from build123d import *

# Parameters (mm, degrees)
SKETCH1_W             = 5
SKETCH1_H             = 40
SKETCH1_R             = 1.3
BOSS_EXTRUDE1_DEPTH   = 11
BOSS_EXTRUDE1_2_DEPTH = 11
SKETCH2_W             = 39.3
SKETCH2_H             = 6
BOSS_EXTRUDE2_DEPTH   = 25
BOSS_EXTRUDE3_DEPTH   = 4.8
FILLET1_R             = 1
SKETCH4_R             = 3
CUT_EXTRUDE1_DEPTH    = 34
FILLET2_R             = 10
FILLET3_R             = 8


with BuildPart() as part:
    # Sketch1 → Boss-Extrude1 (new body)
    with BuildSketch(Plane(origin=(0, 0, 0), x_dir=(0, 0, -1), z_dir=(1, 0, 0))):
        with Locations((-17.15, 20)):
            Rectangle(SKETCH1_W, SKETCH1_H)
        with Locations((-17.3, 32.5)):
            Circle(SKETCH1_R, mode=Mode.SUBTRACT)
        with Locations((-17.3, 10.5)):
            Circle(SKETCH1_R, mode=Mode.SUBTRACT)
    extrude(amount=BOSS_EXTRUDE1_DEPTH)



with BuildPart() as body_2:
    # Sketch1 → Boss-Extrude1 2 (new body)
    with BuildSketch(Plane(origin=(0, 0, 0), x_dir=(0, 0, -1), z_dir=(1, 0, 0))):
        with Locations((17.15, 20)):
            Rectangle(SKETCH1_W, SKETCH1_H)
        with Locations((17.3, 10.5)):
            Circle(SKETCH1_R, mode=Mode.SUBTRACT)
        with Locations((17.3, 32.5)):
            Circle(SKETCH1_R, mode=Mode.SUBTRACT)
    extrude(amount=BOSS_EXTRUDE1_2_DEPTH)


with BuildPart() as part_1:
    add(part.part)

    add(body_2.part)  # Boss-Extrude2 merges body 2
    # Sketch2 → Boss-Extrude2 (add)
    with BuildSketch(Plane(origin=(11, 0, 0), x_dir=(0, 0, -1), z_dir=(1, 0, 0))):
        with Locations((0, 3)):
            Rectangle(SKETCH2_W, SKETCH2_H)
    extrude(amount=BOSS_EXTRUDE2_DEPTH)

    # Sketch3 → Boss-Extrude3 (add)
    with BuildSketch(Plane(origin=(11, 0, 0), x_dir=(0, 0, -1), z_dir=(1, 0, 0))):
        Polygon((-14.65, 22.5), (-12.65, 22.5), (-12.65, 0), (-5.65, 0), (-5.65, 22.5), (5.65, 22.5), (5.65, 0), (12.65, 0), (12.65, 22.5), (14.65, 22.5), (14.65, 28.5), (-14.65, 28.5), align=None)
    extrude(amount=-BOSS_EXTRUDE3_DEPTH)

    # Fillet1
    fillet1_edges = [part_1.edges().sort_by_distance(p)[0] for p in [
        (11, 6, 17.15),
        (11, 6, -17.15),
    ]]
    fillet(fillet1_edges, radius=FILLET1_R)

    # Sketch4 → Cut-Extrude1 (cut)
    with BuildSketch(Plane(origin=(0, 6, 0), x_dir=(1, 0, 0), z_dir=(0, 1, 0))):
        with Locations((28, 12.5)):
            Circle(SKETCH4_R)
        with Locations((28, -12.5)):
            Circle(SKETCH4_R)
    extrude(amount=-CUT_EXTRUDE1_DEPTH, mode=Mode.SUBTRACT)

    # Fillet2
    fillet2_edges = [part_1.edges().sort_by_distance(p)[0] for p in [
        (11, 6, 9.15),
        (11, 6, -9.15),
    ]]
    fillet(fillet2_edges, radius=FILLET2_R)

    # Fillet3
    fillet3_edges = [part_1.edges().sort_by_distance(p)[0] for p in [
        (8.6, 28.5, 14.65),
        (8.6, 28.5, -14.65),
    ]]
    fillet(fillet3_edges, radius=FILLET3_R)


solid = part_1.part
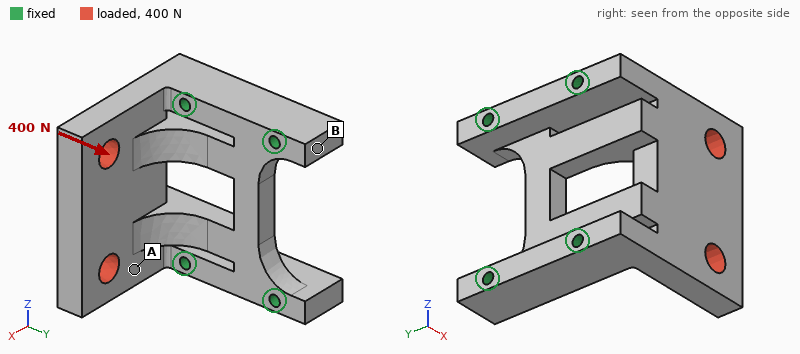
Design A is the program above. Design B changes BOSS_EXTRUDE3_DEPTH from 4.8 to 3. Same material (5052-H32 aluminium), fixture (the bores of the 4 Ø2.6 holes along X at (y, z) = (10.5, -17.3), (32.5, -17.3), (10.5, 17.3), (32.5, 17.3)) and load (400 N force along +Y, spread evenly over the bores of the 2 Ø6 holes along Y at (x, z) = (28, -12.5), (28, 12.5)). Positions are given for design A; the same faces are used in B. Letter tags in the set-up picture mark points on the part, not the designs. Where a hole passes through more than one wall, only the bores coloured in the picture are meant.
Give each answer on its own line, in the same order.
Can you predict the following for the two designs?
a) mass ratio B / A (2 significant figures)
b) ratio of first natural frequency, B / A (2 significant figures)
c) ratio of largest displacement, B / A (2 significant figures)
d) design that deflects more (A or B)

0.93
0.86
1.4
B
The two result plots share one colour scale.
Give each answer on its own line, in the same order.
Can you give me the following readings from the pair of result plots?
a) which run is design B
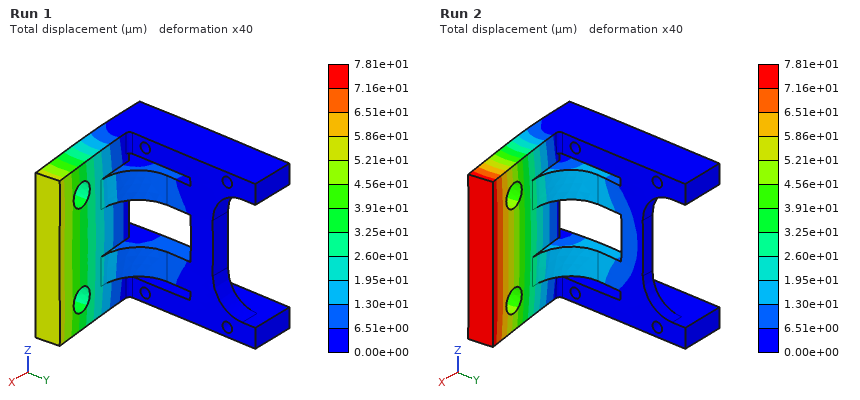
Run 2
